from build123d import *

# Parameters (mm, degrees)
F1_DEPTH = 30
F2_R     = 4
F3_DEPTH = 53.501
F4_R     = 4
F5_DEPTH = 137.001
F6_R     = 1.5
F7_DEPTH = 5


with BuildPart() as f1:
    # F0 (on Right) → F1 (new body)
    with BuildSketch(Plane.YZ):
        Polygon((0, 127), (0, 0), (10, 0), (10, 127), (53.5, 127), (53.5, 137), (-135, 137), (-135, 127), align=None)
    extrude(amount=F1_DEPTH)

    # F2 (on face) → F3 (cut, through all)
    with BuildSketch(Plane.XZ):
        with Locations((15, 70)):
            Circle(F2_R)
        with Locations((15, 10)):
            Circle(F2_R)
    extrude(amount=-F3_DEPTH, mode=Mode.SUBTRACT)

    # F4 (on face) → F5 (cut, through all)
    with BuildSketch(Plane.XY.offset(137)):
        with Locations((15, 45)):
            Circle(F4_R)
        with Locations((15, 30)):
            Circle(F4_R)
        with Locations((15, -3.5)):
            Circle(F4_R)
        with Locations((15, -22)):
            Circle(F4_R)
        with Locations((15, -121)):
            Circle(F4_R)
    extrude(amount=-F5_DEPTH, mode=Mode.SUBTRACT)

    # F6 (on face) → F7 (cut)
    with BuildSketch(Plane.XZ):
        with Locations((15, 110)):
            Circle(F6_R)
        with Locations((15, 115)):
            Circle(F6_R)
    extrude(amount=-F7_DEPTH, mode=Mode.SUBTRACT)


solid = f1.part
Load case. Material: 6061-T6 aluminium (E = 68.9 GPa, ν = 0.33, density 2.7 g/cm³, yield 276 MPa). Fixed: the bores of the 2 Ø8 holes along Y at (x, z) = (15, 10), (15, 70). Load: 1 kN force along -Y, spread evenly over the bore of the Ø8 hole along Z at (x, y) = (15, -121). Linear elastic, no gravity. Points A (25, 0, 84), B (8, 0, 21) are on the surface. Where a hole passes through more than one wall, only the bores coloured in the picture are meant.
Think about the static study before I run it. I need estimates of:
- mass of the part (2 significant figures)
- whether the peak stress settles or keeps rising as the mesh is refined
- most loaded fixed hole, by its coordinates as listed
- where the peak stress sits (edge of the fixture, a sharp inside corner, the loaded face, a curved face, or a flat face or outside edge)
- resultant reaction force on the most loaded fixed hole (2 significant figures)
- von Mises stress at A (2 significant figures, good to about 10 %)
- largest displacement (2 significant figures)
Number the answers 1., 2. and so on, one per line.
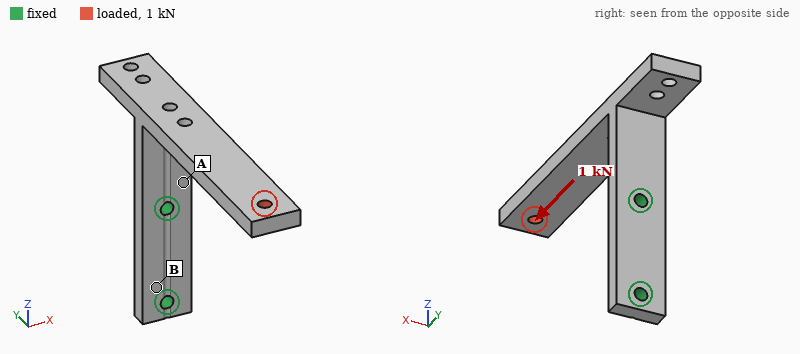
1. 250 g
2. keeps rising
3. (15, 70)
4. edge of the fixture
5. 1.1 kN
6. 91 MPa
7. 1.6 mm
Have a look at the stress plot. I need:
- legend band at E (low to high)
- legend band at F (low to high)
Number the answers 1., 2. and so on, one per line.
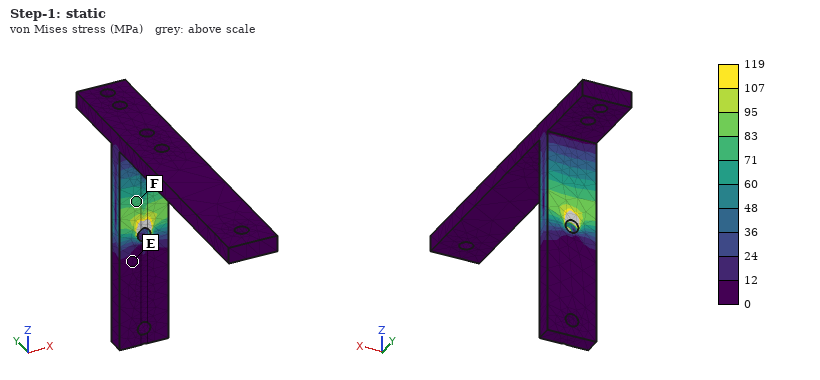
1. 0 to 12 MPa
2. 71 to 83 MPa
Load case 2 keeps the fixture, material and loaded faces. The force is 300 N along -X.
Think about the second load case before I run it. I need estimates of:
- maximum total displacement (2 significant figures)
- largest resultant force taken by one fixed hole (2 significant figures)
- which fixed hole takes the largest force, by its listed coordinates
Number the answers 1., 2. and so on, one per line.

1. 1.6 mm
2. 480 N
3. (15, 70)
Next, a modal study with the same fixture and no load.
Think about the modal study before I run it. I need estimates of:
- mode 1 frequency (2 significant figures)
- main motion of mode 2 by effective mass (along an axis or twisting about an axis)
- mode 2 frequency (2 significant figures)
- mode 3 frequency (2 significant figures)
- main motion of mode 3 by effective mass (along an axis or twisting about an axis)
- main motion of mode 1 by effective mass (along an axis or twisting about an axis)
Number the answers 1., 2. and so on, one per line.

1. 240 Hz
2. along X
3. 340 Hz
4. 820 Hz
5. along Y
6. along Z
